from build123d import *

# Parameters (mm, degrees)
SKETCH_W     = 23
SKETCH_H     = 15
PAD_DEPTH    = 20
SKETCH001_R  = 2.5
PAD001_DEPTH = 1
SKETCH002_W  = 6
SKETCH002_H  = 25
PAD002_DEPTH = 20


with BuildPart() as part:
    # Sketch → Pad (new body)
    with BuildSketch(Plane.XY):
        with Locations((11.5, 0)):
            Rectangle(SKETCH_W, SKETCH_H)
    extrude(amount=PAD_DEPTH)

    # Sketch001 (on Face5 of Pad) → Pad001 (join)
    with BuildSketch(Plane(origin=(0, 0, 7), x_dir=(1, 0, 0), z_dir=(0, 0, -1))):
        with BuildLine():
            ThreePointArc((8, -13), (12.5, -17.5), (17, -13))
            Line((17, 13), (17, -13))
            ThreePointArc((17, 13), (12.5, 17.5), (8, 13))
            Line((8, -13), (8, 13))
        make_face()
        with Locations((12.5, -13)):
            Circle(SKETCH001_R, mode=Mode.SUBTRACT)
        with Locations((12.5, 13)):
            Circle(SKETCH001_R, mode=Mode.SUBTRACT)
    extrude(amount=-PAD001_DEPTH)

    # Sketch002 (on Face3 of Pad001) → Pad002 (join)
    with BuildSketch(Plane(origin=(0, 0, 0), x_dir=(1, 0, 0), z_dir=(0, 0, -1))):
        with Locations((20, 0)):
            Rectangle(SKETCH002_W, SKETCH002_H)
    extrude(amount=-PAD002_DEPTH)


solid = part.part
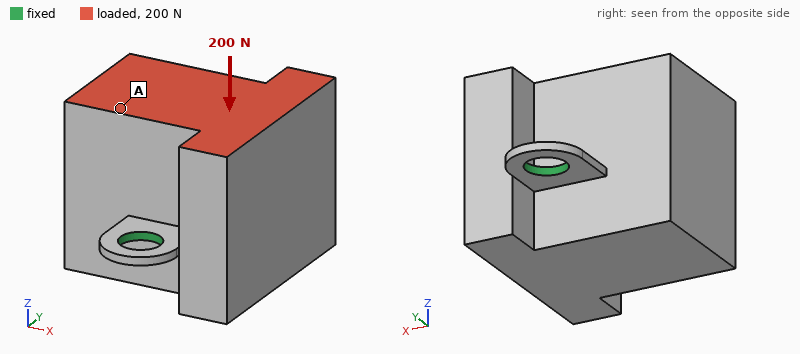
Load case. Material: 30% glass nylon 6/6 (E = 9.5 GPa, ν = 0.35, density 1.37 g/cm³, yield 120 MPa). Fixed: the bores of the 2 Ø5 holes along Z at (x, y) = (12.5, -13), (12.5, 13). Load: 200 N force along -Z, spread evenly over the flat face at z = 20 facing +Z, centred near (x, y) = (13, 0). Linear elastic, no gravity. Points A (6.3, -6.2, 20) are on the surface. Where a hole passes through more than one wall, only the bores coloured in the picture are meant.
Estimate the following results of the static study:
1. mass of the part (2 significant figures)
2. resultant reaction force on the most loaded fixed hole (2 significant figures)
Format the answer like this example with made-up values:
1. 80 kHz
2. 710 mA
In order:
1. 11 g
2. 100 N
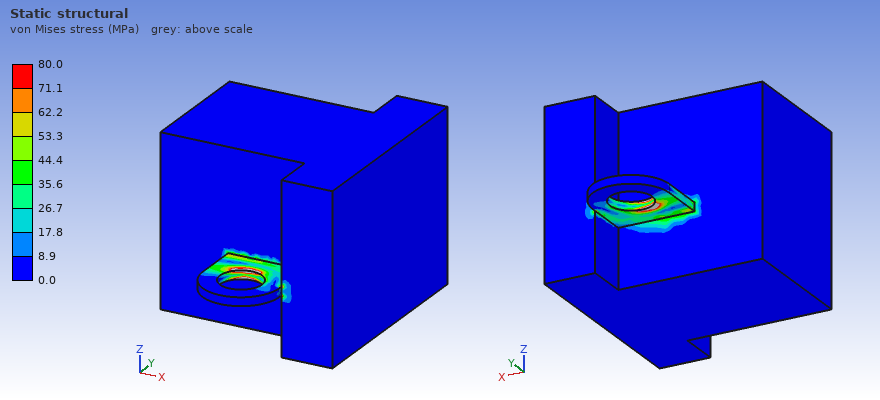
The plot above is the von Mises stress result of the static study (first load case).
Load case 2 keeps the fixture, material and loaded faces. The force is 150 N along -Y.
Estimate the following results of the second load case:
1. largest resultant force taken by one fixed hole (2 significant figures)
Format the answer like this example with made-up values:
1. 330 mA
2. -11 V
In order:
1. 120 N
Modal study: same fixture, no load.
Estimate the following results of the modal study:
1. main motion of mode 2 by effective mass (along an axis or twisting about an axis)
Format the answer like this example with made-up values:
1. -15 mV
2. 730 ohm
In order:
1. along Z
